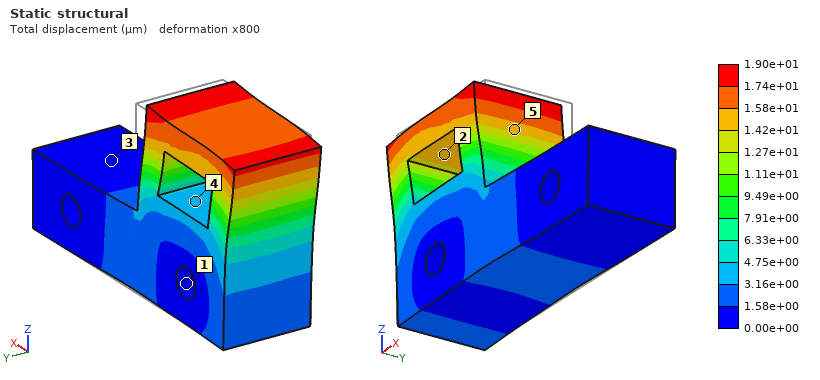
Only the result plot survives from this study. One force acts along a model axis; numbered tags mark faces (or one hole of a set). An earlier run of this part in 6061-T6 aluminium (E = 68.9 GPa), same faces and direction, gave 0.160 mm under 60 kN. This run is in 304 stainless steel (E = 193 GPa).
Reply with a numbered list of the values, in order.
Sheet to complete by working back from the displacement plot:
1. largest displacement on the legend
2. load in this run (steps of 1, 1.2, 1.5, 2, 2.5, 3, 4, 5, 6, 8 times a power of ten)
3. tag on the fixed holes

1. 1.90e+01 µm
2. 20 kN
3. 1
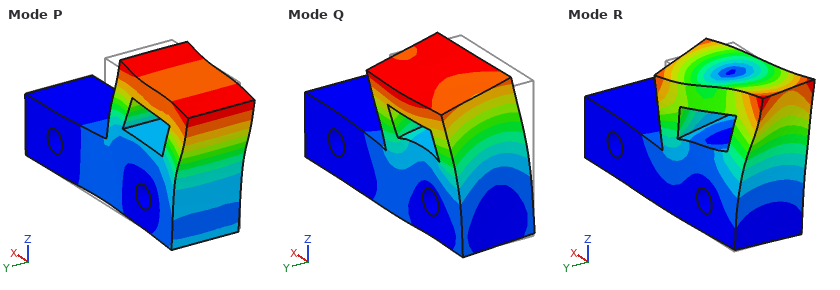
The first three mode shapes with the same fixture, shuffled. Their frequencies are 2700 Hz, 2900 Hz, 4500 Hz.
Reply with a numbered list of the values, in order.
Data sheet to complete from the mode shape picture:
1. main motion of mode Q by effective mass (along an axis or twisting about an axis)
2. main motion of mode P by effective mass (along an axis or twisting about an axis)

1. along Y
2. along X
